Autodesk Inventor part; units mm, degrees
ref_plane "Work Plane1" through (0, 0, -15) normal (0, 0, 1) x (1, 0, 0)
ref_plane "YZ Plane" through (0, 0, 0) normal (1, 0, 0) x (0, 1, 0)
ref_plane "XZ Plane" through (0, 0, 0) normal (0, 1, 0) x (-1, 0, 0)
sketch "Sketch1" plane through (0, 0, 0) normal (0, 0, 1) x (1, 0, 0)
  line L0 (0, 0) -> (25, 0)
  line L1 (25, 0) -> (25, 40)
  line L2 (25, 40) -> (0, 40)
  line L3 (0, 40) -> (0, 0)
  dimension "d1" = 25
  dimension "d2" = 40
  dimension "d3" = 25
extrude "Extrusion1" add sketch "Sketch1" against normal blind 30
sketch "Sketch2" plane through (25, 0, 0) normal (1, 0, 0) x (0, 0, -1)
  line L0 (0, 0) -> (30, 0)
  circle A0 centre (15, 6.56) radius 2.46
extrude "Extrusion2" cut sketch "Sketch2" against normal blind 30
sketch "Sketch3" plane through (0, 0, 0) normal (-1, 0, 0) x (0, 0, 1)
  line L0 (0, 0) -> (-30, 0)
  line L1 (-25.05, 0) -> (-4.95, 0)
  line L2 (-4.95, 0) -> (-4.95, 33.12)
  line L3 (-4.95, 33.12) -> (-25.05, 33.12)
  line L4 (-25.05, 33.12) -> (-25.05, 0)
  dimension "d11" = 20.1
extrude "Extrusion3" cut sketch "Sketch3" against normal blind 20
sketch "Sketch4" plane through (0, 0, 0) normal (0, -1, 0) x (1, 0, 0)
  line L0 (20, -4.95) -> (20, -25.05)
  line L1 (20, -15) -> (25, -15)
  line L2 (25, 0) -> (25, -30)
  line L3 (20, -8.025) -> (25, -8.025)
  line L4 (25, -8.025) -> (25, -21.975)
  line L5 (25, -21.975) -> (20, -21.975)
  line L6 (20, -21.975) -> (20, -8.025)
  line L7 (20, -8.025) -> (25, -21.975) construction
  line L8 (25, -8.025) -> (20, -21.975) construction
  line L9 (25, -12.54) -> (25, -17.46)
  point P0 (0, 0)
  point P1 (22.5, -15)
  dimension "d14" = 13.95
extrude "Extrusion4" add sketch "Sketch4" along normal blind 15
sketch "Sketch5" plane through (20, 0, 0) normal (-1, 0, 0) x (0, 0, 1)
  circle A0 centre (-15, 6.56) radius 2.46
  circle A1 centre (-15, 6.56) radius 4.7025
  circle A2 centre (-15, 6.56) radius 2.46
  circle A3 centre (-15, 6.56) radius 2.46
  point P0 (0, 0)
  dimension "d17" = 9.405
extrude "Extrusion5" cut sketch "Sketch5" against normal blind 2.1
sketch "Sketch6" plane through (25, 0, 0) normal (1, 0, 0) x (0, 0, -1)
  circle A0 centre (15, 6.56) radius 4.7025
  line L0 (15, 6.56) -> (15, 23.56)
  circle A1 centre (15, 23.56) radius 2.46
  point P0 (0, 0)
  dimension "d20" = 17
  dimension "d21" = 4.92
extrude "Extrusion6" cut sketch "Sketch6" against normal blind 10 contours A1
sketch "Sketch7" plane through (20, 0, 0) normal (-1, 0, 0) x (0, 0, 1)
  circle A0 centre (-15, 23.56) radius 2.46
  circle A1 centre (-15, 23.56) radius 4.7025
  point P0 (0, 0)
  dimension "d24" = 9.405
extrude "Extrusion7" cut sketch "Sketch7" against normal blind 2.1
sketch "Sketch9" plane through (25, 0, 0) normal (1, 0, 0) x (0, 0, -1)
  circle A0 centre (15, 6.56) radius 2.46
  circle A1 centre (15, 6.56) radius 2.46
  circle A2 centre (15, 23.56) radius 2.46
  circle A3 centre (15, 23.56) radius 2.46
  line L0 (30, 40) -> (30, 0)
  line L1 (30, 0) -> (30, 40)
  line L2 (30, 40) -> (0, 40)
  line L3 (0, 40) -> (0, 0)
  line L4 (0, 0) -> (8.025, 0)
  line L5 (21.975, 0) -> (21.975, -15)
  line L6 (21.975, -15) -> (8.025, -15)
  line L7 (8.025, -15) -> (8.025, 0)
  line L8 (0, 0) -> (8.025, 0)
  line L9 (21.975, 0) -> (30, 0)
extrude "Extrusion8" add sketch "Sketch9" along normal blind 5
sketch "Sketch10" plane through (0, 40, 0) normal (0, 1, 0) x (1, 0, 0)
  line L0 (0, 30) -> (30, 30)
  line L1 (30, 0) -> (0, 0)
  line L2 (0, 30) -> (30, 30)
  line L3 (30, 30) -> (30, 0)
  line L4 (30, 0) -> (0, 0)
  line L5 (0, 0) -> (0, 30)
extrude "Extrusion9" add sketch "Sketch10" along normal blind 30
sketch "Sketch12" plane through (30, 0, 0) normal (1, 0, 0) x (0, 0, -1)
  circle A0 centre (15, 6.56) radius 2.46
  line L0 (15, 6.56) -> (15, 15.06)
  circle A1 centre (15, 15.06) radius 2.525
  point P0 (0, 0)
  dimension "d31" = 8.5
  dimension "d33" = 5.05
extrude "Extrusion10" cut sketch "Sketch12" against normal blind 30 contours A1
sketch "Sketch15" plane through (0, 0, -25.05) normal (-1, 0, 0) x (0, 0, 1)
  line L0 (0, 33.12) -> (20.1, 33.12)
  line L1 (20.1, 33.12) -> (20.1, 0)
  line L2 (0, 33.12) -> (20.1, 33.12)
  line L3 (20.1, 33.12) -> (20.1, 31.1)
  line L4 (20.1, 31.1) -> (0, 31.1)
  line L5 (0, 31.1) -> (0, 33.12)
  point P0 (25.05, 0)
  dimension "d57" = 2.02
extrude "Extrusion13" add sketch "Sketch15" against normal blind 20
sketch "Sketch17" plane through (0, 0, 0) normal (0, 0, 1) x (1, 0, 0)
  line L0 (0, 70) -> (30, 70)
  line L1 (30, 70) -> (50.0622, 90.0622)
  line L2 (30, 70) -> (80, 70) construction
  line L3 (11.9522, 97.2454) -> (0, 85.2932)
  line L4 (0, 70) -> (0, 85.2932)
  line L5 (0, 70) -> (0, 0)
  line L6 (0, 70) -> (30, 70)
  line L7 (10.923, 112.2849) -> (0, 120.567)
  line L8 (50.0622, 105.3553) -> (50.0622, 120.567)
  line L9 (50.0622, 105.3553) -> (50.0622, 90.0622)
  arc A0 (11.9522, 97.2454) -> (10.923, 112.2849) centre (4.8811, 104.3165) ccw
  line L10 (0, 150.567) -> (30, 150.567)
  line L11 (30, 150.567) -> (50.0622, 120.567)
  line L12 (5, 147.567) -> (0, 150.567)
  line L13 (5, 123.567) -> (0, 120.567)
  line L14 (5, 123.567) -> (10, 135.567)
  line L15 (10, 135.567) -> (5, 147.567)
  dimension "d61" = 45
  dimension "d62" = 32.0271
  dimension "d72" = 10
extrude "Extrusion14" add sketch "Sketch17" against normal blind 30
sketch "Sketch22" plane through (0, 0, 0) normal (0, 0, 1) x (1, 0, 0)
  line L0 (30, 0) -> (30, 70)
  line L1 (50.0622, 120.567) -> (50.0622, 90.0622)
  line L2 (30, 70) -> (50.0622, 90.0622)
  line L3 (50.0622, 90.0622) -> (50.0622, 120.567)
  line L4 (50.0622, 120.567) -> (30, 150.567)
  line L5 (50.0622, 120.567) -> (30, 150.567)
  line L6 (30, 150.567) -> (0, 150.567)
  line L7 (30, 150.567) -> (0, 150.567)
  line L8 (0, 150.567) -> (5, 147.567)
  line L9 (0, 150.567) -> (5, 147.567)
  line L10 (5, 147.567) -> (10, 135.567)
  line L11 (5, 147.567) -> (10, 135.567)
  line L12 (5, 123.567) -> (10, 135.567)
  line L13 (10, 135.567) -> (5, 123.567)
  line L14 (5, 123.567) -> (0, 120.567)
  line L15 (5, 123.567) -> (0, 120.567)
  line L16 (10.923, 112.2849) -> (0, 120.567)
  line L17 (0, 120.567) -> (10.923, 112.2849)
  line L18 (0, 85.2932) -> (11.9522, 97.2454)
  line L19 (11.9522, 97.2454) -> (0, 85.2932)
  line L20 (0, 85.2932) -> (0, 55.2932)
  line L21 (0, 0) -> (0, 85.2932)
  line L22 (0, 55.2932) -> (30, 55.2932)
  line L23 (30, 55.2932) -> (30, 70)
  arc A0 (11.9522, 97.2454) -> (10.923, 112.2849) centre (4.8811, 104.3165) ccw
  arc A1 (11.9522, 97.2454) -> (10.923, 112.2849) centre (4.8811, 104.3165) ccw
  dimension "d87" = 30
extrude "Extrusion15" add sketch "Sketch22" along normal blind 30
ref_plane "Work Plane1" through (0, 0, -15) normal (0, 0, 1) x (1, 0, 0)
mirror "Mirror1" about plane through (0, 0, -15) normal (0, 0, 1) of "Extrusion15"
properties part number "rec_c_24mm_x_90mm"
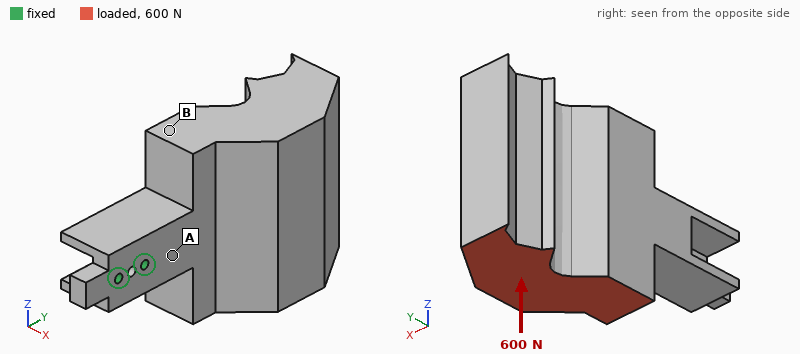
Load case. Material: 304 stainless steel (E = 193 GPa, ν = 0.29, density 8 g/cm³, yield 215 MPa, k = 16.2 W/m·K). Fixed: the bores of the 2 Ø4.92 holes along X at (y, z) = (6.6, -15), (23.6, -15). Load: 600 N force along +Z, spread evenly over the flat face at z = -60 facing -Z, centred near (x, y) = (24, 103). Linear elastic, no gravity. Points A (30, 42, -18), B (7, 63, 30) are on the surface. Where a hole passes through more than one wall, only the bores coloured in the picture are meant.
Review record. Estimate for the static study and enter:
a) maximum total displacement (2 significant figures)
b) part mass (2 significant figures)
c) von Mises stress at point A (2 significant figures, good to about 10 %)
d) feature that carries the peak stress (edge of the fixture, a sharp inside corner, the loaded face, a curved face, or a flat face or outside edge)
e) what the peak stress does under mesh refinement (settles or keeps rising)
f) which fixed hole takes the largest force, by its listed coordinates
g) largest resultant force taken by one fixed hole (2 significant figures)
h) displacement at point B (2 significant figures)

46 µm
2.8 kg
6.6 MPa
edge of the fixture
keeps rising
(23.6, -15)
2.6 kN
19 µm
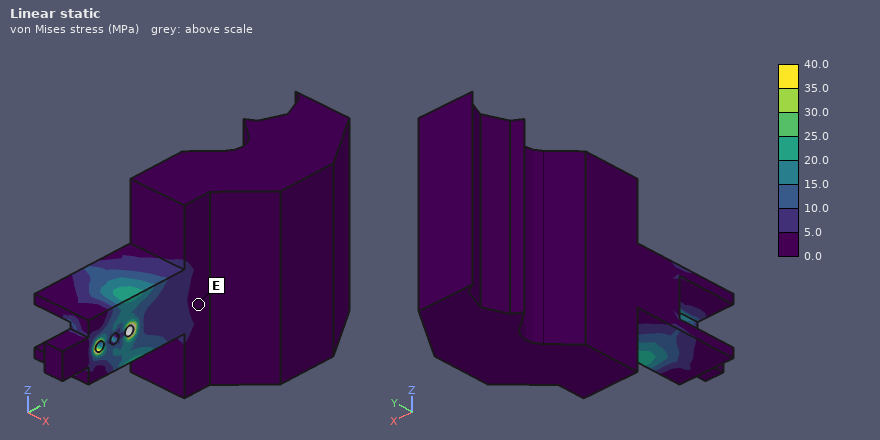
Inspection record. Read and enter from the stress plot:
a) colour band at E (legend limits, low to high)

0.0 to 5.0 MPa
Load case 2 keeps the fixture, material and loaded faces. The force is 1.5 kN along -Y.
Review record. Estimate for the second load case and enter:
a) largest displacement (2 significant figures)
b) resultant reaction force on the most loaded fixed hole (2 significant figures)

73 µm
3.1 kN
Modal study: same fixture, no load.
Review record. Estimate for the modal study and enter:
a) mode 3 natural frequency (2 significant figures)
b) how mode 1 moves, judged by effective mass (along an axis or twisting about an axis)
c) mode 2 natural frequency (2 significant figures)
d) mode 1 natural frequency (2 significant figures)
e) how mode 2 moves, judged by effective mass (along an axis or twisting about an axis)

780 Hz
along X
430 Hz
390 Hz
along Z
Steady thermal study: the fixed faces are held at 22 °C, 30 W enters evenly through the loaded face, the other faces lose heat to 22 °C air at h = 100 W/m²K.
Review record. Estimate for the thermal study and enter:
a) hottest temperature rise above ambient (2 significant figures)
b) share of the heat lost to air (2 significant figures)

26 K
97 %
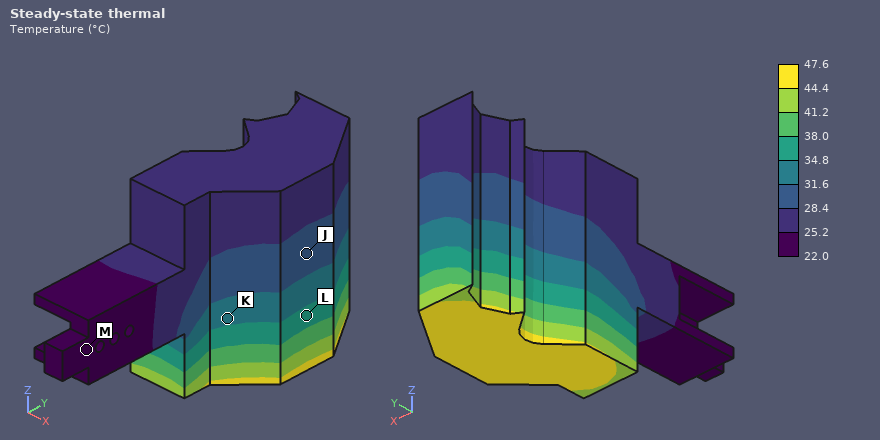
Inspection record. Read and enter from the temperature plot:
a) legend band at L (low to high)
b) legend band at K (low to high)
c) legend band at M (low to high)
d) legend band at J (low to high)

34.8 to 38.0 °C
31.6 to 34.8 °C
22.0 to 25.2 °C
28.4 to 31.6 °C
